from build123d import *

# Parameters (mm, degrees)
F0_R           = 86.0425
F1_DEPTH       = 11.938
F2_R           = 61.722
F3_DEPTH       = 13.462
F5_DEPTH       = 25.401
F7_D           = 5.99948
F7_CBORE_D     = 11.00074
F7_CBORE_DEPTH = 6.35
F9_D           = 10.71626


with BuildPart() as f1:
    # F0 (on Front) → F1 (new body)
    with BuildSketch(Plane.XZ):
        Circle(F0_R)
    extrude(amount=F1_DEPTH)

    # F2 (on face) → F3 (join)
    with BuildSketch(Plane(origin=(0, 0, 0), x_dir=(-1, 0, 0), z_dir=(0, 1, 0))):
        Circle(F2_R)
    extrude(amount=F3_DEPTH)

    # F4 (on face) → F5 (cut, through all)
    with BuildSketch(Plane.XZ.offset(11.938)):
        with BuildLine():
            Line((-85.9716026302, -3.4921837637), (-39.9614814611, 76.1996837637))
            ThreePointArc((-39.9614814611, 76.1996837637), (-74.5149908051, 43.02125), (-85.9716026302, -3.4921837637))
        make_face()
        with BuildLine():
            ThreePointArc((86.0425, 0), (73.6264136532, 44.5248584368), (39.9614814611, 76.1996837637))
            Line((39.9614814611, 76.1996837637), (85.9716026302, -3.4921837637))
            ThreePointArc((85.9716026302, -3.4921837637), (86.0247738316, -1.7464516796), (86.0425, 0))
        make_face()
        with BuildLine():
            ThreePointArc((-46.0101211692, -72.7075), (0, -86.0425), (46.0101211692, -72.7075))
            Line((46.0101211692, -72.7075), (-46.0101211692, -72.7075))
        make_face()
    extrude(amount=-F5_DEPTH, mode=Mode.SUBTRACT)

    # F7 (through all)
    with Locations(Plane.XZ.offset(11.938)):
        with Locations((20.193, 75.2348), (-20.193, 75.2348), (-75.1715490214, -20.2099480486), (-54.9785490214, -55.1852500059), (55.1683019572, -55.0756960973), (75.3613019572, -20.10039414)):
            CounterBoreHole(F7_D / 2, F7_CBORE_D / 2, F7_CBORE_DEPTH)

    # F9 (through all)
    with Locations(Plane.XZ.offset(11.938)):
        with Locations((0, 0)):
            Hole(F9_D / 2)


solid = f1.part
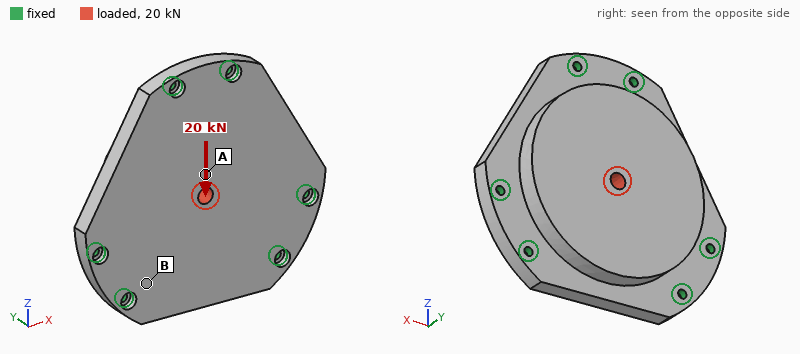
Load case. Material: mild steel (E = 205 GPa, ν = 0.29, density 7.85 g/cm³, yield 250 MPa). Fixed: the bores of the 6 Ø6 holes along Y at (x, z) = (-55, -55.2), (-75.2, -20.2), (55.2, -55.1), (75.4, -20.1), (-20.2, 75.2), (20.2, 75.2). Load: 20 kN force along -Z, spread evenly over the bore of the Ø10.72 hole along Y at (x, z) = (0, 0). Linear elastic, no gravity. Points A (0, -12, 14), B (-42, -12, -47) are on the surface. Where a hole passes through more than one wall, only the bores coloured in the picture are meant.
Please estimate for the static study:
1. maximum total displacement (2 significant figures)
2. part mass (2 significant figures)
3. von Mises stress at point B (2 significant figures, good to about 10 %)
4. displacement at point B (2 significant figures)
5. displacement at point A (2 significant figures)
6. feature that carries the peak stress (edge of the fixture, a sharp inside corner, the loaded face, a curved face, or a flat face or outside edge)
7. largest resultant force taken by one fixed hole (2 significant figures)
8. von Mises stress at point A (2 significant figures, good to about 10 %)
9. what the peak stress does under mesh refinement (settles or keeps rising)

6.2 µm
3.2 kg
6.6 MPa
2.7 µm
4.4 µm
edge of the fixture
4.2 kN
18 MPa
keeps rising
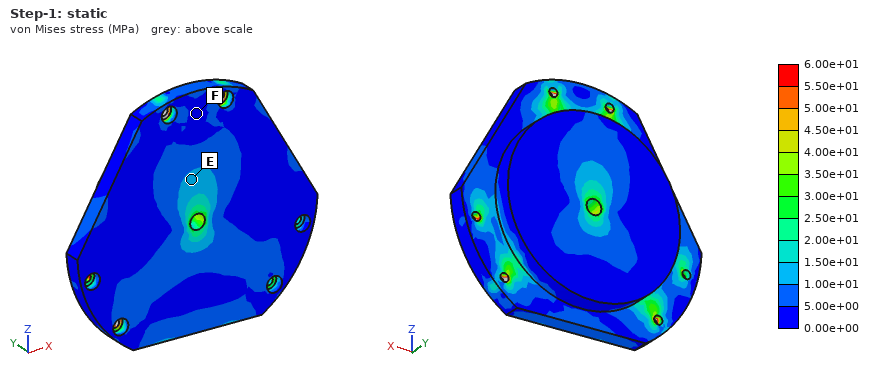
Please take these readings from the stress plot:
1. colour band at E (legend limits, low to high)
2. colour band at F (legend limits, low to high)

1.00e+01 to 1.50e+01 MPa
0.00e+00 to 5.00e+00 MPa
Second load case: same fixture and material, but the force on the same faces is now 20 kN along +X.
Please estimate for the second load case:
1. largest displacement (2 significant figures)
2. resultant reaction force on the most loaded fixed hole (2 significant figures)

6.1 µm
4.2 kN
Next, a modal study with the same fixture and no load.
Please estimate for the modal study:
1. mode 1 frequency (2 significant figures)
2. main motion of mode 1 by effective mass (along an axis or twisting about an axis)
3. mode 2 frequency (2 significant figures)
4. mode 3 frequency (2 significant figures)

3200 Hz
along Y
4800 Hz
4800 Hz
